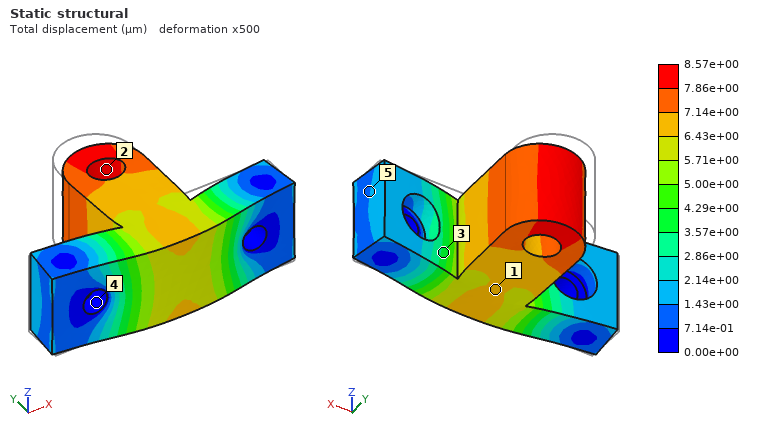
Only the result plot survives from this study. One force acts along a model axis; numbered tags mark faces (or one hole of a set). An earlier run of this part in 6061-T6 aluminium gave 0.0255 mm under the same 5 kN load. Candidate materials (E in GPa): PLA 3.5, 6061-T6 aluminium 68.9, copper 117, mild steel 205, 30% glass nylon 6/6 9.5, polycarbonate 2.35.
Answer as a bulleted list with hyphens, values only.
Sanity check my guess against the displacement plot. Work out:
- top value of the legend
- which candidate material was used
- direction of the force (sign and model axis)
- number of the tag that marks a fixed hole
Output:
- 8.57e+00 µm
- mild steel
- -Y
- 4
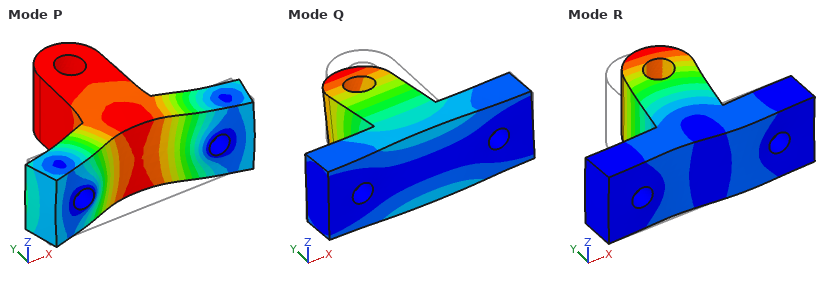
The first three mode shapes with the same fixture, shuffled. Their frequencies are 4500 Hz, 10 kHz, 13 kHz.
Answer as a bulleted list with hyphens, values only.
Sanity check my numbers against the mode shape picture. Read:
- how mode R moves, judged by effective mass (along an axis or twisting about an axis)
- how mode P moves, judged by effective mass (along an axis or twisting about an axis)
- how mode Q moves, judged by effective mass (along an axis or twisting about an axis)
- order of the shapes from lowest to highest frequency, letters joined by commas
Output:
- along X
- along Y
- along Z
- Q, R, P
